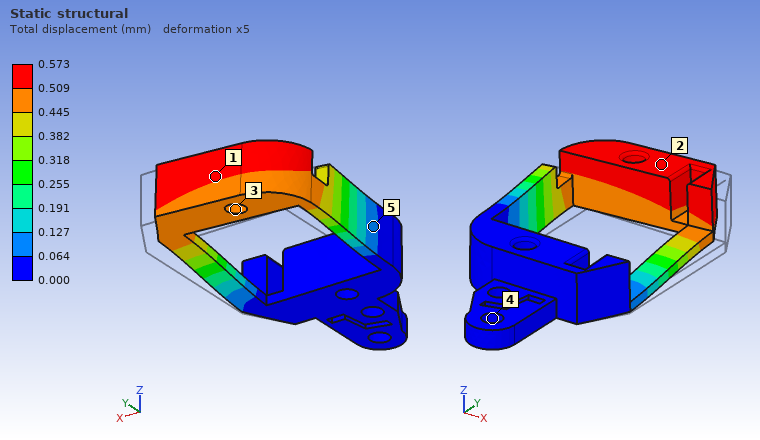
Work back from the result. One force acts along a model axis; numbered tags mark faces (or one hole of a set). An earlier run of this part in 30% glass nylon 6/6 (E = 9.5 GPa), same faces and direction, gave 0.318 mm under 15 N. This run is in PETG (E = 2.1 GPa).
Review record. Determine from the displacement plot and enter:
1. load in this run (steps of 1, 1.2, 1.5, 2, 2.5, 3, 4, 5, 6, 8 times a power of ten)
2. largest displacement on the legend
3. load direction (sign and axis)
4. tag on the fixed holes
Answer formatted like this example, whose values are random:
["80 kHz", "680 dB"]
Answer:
["6 N", "0.573 mm", "-X", "4"]
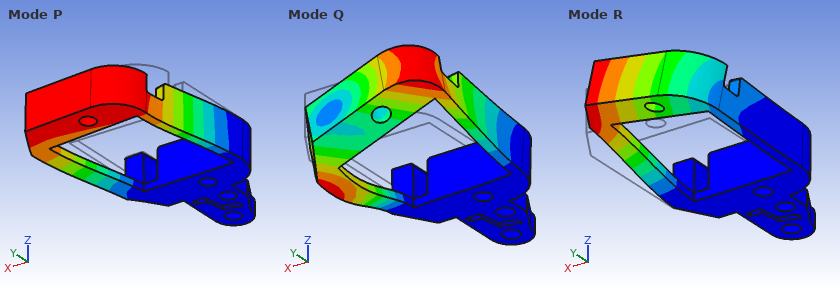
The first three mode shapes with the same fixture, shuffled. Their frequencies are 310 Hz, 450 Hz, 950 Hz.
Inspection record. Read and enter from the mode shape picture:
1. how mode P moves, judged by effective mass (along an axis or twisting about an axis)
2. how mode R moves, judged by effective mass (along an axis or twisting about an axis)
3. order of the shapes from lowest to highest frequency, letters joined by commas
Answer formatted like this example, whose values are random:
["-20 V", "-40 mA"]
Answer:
["along X", "along Z", "R, P, Q"]
